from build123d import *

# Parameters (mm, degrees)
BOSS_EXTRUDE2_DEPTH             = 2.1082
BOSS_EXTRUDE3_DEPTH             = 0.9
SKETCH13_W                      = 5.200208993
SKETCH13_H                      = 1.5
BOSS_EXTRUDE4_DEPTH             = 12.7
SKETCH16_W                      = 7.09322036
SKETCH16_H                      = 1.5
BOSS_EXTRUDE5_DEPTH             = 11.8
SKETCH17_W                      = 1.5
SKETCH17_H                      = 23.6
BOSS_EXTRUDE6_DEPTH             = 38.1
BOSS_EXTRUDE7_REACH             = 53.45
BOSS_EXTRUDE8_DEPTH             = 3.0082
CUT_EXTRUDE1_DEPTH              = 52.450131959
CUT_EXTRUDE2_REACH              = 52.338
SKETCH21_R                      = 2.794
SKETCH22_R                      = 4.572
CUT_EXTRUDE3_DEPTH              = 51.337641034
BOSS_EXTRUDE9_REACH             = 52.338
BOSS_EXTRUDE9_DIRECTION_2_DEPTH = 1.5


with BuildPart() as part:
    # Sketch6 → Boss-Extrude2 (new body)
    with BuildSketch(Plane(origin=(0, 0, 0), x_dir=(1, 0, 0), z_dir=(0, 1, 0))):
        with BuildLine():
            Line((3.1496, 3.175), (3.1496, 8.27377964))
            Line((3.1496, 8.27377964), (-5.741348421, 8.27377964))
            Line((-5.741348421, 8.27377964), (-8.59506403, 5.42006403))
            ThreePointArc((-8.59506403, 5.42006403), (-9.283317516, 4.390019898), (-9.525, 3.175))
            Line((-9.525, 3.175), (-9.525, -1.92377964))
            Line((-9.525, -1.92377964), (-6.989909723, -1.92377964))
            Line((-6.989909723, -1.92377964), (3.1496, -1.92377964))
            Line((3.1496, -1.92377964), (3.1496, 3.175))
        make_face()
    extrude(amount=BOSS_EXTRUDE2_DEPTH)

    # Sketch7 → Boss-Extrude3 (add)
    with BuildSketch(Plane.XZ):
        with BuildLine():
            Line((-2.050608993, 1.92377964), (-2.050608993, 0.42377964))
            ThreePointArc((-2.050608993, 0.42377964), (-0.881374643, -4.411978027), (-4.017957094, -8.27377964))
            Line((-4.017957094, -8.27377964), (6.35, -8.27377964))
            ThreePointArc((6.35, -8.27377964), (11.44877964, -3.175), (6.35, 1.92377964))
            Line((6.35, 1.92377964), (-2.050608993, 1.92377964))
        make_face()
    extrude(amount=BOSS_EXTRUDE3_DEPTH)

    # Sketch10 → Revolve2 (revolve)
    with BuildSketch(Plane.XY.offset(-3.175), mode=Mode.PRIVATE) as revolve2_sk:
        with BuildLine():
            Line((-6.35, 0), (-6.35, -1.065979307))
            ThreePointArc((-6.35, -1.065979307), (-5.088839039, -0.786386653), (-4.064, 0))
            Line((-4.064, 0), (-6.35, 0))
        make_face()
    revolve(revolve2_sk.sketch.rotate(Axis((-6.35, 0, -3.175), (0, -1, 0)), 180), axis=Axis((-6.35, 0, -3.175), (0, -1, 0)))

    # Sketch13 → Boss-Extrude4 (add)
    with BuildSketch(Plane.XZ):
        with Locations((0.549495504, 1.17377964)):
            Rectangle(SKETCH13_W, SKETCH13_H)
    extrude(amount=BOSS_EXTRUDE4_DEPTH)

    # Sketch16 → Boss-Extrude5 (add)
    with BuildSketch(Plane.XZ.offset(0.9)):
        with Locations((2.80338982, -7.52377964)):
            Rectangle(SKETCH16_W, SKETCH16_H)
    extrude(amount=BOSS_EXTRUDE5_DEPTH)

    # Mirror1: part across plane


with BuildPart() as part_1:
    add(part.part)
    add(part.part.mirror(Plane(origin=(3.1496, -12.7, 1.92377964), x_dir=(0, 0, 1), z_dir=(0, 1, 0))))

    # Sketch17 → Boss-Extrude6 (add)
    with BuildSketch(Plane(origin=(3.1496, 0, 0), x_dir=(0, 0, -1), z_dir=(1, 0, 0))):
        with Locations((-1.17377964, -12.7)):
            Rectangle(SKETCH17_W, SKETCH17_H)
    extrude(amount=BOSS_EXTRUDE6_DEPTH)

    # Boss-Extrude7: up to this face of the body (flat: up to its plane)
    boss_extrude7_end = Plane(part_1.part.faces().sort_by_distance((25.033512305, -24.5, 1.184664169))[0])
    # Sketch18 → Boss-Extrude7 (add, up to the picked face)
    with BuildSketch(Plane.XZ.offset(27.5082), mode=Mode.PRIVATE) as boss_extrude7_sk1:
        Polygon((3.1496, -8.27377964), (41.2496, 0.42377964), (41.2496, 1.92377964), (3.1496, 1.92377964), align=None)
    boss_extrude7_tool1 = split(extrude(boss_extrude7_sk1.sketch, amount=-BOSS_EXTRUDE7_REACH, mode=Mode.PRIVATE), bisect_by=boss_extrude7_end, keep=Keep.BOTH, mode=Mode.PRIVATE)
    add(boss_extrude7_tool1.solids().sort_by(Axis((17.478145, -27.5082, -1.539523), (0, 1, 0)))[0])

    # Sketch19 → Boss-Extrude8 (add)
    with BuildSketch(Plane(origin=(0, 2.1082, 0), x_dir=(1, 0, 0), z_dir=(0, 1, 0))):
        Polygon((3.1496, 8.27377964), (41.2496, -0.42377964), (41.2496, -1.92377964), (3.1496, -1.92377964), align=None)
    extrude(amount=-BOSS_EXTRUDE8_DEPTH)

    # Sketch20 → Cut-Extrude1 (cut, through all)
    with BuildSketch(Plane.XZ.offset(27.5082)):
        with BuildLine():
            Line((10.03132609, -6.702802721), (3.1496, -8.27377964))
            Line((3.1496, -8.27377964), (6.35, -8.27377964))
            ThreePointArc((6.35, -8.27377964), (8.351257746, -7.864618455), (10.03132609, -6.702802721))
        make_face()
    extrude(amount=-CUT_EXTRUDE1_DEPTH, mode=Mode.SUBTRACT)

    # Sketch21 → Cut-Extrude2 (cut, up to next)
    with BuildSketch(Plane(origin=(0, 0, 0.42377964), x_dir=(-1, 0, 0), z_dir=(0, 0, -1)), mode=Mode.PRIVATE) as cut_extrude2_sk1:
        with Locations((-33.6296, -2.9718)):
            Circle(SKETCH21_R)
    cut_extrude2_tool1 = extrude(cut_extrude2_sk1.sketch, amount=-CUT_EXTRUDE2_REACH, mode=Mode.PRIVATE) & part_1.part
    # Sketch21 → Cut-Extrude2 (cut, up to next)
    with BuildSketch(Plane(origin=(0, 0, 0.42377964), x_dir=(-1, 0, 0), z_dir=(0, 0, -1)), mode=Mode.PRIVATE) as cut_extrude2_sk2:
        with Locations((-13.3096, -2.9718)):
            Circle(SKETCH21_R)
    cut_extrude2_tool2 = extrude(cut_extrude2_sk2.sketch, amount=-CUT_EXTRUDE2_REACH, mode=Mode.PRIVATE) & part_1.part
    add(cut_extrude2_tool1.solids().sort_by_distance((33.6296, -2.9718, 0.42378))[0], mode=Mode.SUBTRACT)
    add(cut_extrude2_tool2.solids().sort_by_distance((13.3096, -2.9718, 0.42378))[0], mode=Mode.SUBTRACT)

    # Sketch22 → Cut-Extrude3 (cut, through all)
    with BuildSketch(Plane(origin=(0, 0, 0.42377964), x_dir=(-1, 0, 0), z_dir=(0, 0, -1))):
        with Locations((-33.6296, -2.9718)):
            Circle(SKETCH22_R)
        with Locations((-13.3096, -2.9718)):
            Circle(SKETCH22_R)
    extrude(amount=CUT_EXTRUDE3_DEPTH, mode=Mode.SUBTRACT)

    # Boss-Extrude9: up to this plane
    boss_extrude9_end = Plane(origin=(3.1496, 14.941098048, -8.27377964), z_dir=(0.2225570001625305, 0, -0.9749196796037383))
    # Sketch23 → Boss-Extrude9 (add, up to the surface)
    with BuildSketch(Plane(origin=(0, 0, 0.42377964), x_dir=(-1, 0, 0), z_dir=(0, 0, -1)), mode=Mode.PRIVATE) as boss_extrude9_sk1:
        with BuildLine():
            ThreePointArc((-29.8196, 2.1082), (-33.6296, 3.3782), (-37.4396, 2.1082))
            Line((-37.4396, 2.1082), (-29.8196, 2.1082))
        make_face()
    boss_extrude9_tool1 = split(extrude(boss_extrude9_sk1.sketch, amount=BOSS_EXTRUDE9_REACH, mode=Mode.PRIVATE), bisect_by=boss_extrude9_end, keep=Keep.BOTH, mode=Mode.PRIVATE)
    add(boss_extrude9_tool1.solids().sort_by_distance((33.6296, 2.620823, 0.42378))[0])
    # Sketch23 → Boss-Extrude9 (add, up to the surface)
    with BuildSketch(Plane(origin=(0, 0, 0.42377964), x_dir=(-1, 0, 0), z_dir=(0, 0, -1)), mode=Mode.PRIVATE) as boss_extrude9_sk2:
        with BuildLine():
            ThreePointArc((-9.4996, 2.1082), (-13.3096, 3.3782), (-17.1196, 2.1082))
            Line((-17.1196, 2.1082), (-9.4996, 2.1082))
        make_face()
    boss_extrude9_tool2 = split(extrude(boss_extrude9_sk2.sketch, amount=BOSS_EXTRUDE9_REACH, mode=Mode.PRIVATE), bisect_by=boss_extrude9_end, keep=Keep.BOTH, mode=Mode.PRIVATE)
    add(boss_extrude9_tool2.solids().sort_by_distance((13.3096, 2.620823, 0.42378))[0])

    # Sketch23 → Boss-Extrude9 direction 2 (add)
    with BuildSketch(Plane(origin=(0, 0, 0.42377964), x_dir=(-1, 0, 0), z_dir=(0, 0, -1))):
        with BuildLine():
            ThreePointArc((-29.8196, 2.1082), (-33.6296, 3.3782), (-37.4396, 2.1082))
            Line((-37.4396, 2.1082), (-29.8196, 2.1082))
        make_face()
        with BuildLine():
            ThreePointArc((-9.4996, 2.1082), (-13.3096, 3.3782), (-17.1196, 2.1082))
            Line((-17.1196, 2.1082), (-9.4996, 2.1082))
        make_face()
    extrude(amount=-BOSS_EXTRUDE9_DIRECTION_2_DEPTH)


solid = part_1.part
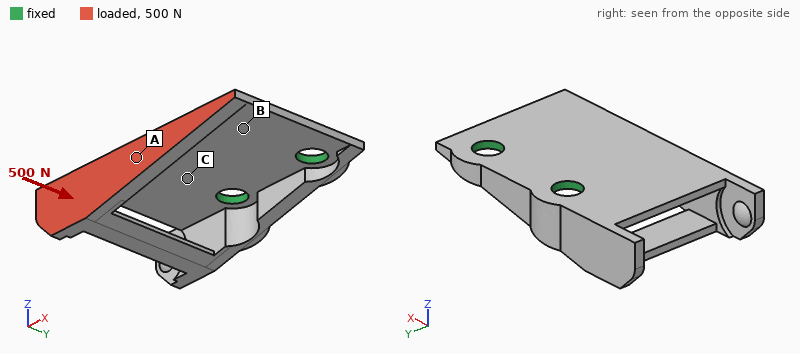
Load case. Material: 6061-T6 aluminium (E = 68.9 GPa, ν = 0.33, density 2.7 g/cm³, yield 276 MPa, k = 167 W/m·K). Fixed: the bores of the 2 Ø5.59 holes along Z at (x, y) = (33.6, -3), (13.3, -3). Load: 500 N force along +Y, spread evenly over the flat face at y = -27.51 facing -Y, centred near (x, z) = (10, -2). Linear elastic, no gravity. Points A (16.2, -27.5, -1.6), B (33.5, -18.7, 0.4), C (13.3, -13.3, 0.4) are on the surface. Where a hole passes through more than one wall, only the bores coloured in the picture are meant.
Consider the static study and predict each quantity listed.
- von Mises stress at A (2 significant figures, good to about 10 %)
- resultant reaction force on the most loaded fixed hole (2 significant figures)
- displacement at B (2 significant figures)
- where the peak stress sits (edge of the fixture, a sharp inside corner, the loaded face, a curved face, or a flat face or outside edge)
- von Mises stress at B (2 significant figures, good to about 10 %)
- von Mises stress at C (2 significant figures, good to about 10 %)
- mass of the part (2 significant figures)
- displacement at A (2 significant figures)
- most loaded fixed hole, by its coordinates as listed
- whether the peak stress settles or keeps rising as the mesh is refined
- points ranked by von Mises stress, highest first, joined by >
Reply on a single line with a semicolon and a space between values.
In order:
10 MPa; 510 N; 0.055 mm; edge of the fixture; 23 MPa; 34 MPa; 9.7 g; 0.14 mm; (13.3, -3); keeps rising; C > B > A
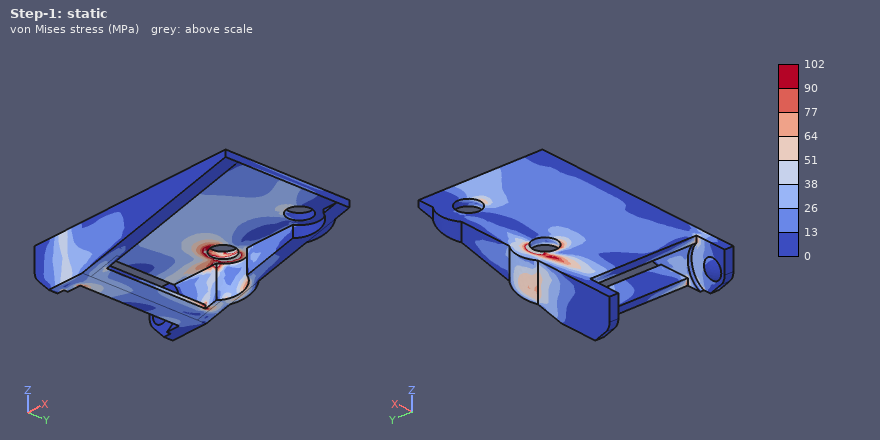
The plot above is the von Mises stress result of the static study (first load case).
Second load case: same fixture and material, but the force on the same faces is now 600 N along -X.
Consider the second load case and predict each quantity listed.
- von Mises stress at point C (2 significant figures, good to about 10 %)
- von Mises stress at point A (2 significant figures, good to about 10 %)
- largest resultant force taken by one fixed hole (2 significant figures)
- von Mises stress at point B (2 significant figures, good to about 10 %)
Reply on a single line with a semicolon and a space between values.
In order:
57 MPa; 28 MPa; 670 N; 51 MPa
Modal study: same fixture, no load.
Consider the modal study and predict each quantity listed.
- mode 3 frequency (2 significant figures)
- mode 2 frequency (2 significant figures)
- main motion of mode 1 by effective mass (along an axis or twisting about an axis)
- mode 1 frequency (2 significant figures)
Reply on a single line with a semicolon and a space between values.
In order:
6800 Hz; 3000 Hz; along Z; 1700 Hz
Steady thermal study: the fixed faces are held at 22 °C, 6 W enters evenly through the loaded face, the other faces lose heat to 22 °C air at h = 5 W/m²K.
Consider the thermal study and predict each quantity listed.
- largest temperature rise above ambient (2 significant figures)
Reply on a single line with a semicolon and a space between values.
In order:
17 K
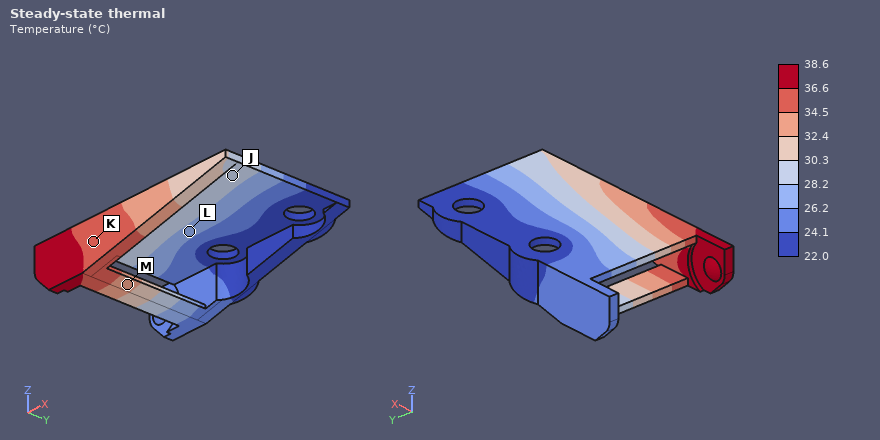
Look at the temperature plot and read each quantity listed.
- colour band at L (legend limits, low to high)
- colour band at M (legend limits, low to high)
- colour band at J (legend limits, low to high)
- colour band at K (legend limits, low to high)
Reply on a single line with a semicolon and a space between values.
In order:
26.2 to 28.2 °C; 32.4 to 34.5 °C; 28.2 to 30.3 °C; 34.5 to 36.6 °C
